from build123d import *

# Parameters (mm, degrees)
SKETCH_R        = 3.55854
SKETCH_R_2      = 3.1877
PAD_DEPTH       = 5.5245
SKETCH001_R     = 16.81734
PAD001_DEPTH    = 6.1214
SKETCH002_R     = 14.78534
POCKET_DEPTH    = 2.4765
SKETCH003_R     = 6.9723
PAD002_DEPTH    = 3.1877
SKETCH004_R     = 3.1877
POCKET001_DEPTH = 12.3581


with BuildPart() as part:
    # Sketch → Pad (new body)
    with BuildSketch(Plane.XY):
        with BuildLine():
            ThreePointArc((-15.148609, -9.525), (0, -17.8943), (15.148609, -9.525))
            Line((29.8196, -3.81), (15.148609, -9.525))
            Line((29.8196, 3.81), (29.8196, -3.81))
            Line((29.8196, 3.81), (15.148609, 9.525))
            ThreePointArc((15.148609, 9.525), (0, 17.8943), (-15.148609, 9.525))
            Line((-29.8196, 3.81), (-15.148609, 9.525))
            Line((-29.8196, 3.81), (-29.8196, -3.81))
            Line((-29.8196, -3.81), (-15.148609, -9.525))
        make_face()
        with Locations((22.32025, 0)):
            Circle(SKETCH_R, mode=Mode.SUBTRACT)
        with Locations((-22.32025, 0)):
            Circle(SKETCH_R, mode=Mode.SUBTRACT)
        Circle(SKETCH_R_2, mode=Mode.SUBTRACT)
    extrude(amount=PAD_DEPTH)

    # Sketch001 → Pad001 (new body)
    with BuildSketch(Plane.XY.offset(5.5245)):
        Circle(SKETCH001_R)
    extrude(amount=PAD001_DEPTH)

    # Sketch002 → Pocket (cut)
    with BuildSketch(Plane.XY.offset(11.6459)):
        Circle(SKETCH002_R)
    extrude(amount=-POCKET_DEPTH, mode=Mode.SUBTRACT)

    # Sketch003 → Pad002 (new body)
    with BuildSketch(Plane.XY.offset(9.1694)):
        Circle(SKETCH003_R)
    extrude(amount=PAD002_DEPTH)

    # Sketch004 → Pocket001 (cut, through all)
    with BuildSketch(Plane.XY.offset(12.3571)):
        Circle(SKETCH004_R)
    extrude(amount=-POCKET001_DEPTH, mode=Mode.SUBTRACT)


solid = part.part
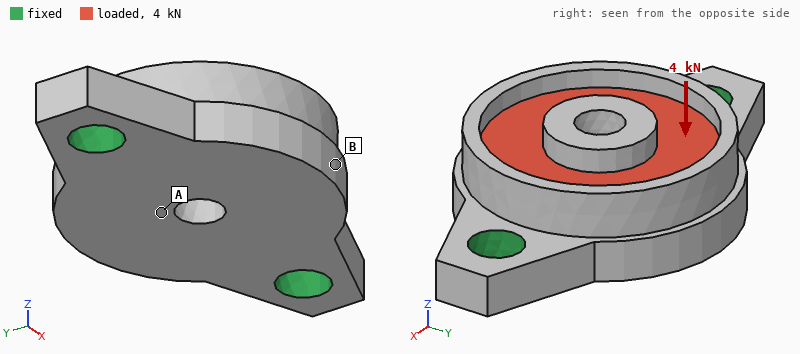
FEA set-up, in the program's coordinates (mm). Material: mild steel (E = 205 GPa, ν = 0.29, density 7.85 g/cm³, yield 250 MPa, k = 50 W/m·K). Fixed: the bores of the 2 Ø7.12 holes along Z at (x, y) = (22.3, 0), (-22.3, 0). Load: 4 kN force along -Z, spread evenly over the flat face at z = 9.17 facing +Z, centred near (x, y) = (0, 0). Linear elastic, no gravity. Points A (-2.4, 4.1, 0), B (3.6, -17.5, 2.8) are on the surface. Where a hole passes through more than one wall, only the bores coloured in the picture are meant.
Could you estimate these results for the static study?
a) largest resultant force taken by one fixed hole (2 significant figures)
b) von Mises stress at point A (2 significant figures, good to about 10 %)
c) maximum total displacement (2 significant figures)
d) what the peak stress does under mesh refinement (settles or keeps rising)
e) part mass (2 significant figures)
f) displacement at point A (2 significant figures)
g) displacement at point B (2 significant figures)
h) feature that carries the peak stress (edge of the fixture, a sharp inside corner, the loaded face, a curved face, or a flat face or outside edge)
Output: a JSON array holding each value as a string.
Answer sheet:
["2.4 kN", "33 MPa", "10.0 µm", "keeps rising", "84 g", "7.6 µm", "9.7 µm", "edge of the fixture"]
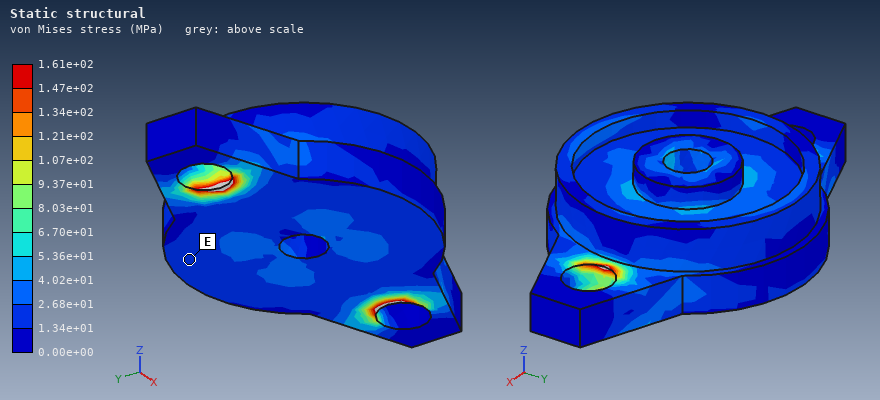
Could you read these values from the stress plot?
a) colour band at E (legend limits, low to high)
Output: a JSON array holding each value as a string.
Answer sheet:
["1.34e+01 to 2.68e+01 MPa"]
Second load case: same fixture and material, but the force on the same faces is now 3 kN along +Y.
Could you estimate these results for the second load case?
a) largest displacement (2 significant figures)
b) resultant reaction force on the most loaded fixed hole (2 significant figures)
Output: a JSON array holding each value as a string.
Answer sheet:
["17 µm", "1.5 kN"]
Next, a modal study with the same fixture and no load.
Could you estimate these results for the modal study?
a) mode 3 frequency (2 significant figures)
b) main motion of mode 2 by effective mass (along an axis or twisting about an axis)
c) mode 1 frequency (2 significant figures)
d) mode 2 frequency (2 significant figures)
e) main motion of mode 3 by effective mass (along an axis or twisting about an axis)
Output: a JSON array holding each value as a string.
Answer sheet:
["23 kHz", "along Z", "9400 Hz", "14 kHz", "along Y"]
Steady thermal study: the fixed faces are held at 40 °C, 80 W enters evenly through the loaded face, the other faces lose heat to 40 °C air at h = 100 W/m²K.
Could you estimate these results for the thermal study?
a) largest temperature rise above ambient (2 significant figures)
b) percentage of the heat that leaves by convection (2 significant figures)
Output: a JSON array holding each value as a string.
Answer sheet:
["73 K", "23 %"]
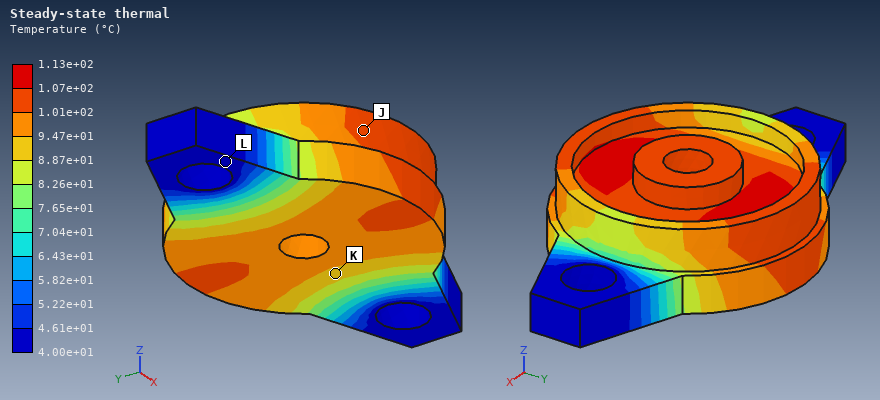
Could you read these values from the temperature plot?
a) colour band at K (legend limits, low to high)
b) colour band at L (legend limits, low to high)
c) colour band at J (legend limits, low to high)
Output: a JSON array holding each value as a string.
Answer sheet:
["8.87e+01 to 9.47e+01 °C", "4.00e+01 to 4.61e+01 °C", "1.01e+02 to 1.07e+02 °C"]
